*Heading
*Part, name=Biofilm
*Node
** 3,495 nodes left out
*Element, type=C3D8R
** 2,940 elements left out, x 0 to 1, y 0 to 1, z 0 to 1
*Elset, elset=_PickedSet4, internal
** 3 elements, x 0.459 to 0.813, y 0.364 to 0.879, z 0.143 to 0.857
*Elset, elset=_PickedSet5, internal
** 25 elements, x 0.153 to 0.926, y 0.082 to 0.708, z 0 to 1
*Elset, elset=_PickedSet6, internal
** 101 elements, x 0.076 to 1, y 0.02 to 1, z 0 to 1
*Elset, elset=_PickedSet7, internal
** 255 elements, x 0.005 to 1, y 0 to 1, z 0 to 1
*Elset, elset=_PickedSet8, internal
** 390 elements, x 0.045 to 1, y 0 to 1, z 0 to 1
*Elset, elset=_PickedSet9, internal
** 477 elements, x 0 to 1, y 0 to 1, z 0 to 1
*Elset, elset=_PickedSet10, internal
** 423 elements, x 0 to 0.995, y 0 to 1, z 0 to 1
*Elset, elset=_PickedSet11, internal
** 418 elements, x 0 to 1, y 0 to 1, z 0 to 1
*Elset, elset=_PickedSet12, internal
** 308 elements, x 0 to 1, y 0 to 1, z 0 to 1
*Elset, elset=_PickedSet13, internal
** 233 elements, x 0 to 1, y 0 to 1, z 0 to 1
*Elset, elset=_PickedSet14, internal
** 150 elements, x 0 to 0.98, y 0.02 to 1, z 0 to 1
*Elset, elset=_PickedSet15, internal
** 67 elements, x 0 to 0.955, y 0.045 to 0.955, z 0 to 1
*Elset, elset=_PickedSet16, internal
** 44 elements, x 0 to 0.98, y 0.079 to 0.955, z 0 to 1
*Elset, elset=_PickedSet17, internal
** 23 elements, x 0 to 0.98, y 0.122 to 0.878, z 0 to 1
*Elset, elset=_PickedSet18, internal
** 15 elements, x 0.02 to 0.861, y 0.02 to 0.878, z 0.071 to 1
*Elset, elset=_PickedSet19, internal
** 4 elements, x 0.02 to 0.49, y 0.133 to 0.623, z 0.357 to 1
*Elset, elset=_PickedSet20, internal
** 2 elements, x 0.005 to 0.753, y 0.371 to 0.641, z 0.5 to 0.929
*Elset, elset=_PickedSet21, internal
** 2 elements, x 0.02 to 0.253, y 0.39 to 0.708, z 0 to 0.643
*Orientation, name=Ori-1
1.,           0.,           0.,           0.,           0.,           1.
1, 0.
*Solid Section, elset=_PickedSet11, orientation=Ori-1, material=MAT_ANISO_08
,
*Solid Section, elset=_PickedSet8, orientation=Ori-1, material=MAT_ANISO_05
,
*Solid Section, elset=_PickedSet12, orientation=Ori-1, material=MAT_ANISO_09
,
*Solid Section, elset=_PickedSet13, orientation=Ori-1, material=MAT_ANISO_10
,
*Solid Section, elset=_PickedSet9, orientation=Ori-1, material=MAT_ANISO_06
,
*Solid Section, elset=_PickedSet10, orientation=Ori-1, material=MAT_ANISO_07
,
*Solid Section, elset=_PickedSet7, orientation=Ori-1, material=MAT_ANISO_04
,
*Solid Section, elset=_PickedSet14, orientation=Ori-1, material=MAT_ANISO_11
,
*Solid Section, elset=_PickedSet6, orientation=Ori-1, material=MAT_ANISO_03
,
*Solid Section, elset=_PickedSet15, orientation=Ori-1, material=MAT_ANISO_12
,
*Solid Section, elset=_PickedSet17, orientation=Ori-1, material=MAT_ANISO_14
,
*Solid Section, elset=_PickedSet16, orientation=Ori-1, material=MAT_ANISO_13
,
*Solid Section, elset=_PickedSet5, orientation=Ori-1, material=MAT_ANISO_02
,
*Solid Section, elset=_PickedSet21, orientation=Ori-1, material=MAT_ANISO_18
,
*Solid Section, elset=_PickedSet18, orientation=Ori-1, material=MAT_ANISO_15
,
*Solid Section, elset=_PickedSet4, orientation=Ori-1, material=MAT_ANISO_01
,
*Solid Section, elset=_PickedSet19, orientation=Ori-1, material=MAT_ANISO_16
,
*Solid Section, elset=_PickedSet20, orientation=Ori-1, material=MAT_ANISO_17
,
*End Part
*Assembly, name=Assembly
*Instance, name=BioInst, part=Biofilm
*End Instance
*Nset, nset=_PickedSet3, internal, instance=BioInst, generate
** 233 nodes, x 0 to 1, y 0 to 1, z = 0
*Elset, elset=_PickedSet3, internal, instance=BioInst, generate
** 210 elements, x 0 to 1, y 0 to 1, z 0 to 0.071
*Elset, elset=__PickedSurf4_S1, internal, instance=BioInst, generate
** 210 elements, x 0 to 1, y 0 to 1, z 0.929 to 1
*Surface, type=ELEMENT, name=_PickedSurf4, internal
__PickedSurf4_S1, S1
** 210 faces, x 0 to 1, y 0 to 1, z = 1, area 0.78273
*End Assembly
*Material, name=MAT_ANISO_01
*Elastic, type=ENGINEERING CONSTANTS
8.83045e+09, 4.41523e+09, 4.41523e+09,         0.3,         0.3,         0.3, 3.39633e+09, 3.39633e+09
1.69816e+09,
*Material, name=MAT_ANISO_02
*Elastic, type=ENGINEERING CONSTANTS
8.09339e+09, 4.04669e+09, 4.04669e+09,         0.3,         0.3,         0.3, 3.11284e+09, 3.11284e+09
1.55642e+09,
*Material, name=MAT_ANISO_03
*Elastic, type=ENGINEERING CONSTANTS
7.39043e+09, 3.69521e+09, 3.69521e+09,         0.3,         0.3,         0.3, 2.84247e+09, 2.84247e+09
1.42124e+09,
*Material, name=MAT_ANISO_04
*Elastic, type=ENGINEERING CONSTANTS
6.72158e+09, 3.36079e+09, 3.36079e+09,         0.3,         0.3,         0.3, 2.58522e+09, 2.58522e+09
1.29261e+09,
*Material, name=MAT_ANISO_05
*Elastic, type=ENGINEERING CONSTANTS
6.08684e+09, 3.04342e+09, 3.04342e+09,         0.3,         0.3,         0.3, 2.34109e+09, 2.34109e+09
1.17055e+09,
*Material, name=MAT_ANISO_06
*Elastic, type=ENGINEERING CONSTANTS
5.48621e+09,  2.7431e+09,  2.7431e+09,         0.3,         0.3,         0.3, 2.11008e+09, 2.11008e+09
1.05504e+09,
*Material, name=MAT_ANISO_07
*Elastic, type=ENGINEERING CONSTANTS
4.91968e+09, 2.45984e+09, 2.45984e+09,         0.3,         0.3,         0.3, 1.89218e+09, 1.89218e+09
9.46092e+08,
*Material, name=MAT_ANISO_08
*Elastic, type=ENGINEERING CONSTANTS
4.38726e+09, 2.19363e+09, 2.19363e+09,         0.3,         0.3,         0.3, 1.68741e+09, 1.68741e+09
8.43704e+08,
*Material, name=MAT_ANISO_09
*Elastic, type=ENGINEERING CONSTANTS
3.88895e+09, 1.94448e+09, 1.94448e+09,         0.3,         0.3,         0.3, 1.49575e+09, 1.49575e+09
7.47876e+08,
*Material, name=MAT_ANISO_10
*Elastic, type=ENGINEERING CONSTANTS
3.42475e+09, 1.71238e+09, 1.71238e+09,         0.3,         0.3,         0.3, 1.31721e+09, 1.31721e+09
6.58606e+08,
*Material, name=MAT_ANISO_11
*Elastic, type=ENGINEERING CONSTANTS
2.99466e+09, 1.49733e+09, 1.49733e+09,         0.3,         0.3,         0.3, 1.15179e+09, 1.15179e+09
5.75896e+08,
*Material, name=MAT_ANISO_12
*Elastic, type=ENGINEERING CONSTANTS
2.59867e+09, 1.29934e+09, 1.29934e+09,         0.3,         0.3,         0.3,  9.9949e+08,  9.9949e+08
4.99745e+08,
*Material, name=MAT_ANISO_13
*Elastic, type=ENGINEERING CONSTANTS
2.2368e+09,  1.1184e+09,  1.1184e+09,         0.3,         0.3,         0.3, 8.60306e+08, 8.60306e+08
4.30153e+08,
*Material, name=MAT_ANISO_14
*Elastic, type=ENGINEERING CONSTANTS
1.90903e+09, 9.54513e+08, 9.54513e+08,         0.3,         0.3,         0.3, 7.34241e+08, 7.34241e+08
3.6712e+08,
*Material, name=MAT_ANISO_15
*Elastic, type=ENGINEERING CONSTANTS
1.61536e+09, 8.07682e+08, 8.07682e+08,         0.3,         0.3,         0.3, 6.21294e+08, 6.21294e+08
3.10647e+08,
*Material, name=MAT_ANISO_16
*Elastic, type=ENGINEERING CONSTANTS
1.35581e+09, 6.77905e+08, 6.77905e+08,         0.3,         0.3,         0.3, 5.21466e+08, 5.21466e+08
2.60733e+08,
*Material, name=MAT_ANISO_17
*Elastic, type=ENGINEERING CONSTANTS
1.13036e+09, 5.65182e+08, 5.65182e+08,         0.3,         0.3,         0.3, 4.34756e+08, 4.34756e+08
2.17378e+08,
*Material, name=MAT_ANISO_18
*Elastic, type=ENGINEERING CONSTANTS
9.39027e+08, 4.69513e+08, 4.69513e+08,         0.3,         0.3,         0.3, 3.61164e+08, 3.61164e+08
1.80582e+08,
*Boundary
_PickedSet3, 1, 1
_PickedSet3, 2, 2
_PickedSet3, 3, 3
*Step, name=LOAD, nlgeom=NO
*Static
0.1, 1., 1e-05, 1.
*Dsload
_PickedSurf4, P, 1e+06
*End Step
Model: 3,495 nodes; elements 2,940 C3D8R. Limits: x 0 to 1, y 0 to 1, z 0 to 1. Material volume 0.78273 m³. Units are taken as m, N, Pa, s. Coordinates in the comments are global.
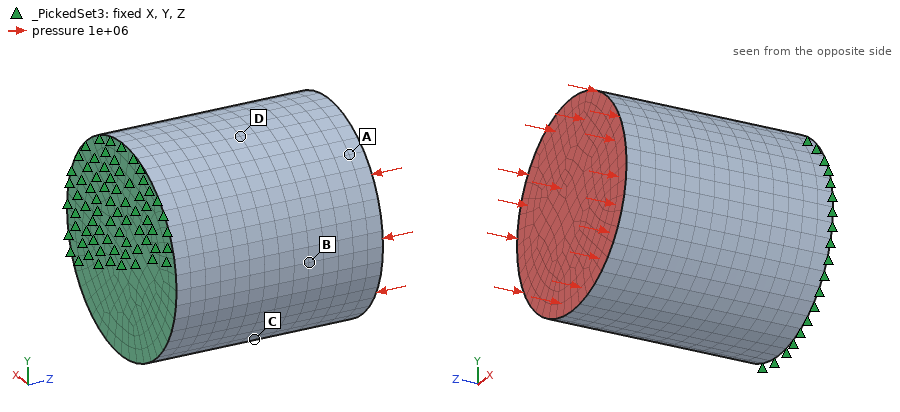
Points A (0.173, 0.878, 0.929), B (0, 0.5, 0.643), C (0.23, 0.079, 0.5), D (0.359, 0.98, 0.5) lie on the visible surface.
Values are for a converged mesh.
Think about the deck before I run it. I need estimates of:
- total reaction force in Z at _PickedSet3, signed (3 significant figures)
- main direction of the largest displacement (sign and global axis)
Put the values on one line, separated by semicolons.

7.83e+05 N; -Z
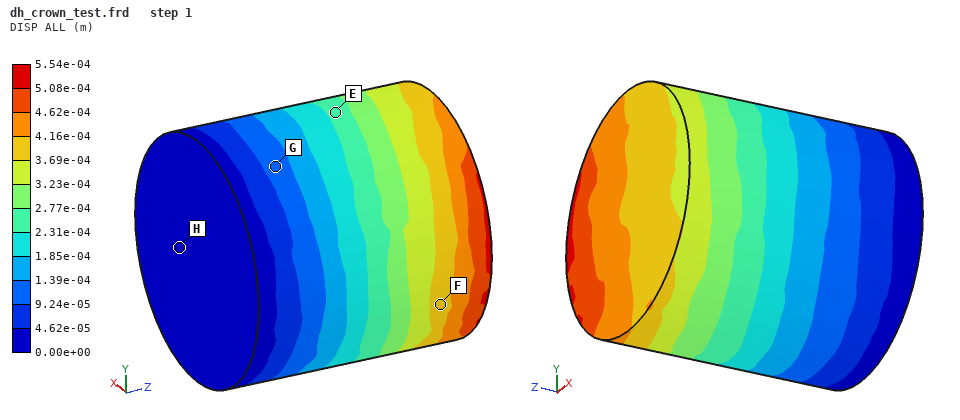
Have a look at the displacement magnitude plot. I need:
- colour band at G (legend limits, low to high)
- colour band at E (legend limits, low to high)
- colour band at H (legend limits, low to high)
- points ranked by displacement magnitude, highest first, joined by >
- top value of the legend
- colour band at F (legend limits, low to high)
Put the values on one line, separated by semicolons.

9.24e-05 to 1.39e-04 m; 2.31e-04 to 2.77e-04 m; 0.00e+00 to 4.62e-05 m; F > E > G > H; 5.54e-04 m; 3.69e-04 to 4.16e-04 m
